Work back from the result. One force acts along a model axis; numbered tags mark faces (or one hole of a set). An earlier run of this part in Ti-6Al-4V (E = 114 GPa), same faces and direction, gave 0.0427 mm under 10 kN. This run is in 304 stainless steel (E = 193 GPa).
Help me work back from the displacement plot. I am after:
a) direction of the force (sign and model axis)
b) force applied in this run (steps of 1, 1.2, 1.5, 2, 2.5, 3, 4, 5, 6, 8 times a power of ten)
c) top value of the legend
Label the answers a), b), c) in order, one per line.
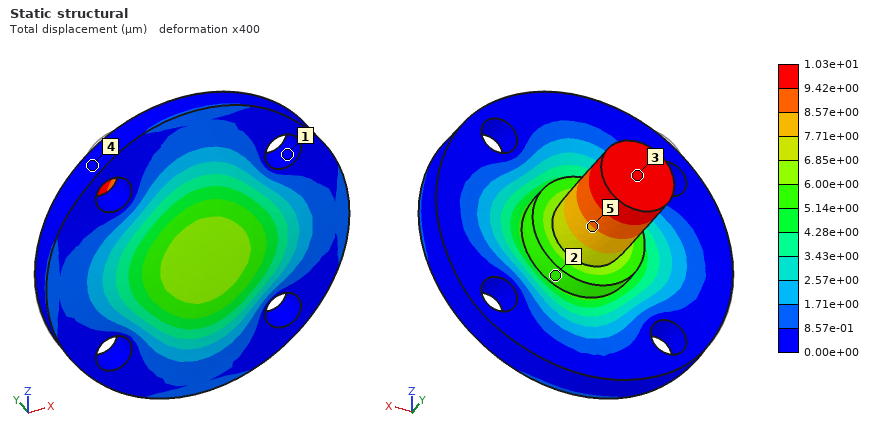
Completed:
a) -Y
b) 4 kN
c) 1.03e+01 µm
